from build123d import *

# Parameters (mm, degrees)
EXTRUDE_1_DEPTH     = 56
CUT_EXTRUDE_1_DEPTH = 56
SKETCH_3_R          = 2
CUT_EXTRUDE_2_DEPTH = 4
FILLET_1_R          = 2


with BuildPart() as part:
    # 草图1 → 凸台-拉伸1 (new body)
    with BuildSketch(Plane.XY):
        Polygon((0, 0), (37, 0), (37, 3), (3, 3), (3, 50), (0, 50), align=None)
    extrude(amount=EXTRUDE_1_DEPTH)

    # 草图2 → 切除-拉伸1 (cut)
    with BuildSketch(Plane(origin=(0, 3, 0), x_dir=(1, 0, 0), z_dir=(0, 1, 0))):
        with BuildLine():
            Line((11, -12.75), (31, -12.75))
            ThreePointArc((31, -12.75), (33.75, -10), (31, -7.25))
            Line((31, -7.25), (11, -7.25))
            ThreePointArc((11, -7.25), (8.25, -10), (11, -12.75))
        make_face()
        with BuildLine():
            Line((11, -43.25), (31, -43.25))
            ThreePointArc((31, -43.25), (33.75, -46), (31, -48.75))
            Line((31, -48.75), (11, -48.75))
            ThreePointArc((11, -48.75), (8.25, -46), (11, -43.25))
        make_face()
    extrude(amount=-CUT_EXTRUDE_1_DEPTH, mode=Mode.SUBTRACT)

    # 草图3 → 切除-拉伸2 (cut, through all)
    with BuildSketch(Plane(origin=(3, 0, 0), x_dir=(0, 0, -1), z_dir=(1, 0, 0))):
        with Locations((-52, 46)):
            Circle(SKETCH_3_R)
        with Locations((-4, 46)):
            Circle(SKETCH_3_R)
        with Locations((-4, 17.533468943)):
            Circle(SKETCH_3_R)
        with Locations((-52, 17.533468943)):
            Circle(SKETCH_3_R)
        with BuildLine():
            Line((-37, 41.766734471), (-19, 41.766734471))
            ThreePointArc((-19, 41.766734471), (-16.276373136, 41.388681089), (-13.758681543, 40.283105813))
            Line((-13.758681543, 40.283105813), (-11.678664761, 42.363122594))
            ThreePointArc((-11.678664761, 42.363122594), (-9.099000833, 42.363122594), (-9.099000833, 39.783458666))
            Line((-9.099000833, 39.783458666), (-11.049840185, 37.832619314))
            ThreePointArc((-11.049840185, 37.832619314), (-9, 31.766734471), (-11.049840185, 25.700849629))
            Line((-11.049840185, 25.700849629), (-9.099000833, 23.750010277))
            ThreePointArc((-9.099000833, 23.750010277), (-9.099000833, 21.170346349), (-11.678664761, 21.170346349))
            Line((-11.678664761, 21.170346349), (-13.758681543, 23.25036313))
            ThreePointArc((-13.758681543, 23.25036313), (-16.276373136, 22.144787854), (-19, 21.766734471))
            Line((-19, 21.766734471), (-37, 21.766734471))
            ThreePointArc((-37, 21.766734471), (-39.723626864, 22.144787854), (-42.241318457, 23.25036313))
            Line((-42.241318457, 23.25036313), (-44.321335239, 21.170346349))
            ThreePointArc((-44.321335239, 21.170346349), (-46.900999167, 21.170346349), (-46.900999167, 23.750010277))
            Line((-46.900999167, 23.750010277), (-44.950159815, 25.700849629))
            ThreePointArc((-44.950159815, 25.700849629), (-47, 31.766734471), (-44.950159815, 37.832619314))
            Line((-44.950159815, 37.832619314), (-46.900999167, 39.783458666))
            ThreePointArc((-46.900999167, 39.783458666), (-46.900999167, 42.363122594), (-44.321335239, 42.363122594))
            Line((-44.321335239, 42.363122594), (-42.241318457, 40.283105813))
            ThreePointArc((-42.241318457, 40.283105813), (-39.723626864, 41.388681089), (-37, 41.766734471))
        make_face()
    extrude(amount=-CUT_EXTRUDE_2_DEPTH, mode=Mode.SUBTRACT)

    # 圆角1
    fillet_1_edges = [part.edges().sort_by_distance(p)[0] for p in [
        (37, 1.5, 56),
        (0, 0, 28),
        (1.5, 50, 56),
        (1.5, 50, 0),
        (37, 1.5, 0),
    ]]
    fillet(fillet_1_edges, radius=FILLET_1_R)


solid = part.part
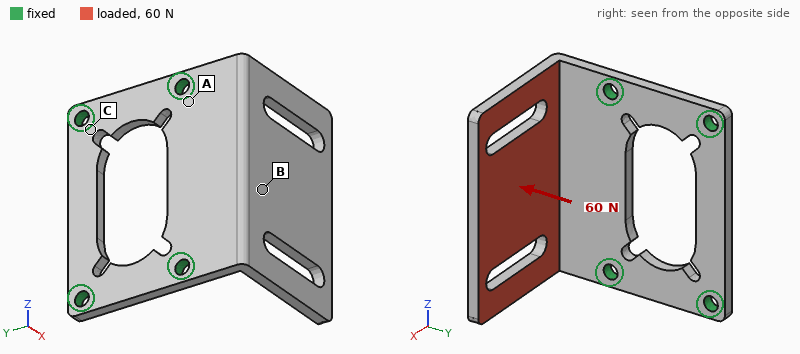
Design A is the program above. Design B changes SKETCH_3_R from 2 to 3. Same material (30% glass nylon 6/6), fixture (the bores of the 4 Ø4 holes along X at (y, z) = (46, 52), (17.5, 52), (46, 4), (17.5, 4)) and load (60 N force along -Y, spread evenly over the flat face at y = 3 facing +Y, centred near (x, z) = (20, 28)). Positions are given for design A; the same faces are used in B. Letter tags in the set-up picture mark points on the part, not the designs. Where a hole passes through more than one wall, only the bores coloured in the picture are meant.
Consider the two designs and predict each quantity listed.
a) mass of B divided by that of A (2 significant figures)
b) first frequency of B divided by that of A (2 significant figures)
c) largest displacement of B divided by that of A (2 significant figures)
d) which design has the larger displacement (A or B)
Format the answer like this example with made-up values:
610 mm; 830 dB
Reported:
0.98; 1.1; 0.90; A
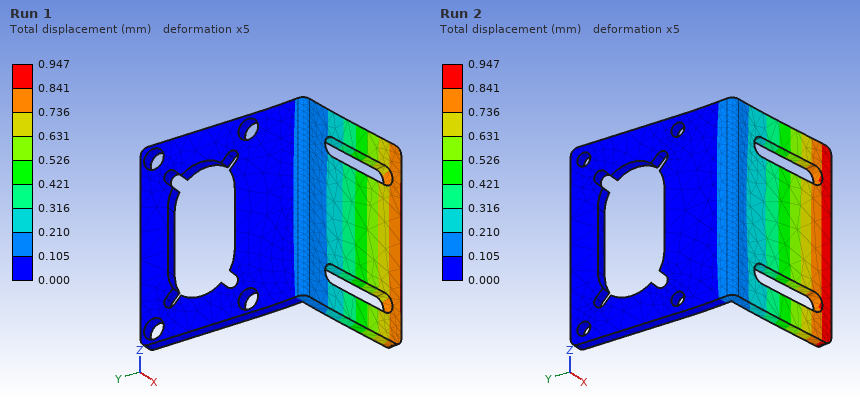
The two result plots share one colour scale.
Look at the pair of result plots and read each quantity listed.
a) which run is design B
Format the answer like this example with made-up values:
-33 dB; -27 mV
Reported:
Run 1
